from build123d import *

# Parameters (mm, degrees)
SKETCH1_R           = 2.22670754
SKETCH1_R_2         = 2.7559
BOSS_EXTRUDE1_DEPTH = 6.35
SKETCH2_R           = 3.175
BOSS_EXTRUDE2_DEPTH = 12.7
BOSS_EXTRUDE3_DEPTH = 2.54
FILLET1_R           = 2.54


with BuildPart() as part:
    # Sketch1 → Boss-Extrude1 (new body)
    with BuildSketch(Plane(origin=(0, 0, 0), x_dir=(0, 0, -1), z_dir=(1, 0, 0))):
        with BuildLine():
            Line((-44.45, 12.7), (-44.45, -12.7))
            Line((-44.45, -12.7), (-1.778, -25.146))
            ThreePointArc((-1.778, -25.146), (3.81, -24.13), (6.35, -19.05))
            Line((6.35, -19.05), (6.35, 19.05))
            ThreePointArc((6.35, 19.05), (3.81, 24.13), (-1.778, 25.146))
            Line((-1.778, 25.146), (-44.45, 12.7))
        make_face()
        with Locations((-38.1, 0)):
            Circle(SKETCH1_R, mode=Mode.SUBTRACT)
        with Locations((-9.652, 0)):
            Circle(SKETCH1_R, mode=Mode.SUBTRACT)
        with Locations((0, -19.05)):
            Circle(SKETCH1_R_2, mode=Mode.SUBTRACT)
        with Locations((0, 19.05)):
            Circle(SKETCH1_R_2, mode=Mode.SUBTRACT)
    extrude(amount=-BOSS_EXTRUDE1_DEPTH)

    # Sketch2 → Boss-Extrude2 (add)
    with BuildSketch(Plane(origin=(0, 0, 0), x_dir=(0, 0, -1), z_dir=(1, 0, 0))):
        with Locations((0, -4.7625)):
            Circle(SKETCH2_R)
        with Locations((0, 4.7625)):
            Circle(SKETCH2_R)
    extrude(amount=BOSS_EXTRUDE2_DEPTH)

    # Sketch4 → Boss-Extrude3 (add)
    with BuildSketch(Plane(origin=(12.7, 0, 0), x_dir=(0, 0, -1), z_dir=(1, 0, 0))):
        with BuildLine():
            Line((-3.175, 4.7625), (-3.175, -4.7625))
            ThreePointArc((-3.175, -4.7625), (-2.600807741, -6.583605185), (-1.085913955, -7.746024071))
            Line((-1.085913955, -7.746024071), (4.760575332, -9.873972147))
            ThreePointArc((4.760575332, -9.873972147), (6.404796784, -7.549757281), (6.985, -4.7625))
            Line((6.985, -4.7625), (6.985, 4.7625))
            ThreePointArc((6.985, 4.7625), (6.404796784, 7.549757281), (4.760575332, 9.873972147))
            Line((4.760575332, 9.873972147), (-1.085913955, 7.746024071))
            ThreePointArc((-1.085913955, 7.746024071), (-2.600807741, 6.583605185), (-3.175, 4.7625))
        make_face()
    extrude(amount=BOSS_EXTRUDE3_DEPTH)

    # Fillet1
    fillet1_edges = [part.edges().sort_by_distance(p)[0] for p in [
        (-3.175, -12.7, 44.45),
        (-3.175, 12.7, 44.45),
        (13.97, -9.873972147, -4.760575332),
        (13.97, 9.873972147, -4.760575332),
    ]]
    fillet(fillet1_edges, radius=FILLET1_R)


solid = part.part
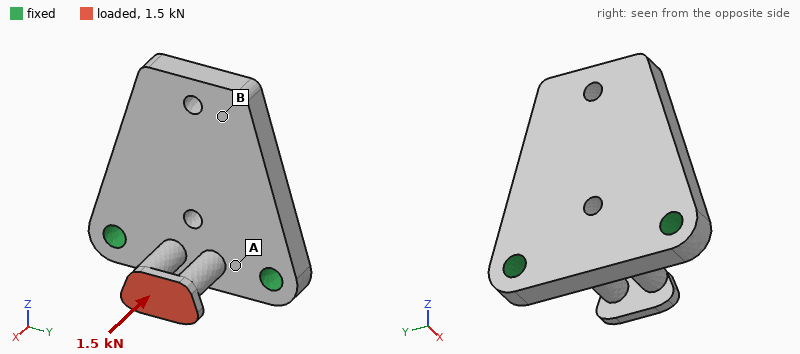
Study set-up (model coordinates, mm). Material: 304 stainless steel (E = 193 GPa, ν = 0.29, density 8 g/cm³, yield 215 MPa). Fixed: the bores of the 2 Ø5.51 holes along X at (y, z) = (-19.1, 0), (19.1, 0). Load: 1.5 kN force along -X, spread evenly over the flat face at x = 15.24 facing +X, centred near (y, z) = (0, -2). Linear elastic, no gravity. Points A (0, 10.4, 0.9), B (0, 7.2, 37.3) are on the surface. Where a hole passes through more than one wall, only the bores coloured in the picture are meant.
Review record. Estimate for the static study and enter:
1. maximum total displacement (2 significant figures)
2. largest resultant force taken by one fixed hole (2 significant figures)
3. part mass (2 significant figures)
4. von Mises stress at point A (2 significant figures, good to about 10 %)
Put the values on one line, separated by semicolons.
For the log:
31 µm; 760 N; 110 g; 21 MPa
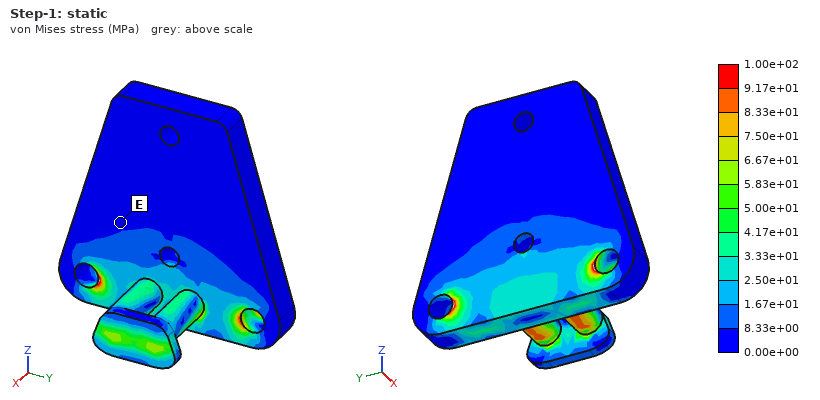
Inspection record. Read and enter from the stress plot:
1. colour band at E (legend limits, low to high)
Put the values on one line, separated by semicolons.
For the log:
0.00e+00 to 8.33e+00 MPa
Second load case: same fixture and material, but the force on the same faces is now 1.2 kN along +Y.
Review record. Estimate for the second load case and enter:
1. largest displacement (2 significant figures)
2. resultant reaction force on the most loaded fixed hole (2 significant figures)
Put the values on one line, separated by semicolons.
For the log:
37 µm; 1000 N
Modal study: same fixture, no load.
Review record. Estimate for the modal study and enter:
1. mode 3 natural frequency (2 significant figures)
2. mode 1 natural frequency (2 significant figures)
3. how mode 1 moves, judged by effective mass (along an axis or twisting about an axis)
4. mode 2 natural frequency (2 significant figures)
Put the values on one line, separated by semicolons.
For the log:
9200 Hz; 2800 Hz; along X; 9100 Hz
